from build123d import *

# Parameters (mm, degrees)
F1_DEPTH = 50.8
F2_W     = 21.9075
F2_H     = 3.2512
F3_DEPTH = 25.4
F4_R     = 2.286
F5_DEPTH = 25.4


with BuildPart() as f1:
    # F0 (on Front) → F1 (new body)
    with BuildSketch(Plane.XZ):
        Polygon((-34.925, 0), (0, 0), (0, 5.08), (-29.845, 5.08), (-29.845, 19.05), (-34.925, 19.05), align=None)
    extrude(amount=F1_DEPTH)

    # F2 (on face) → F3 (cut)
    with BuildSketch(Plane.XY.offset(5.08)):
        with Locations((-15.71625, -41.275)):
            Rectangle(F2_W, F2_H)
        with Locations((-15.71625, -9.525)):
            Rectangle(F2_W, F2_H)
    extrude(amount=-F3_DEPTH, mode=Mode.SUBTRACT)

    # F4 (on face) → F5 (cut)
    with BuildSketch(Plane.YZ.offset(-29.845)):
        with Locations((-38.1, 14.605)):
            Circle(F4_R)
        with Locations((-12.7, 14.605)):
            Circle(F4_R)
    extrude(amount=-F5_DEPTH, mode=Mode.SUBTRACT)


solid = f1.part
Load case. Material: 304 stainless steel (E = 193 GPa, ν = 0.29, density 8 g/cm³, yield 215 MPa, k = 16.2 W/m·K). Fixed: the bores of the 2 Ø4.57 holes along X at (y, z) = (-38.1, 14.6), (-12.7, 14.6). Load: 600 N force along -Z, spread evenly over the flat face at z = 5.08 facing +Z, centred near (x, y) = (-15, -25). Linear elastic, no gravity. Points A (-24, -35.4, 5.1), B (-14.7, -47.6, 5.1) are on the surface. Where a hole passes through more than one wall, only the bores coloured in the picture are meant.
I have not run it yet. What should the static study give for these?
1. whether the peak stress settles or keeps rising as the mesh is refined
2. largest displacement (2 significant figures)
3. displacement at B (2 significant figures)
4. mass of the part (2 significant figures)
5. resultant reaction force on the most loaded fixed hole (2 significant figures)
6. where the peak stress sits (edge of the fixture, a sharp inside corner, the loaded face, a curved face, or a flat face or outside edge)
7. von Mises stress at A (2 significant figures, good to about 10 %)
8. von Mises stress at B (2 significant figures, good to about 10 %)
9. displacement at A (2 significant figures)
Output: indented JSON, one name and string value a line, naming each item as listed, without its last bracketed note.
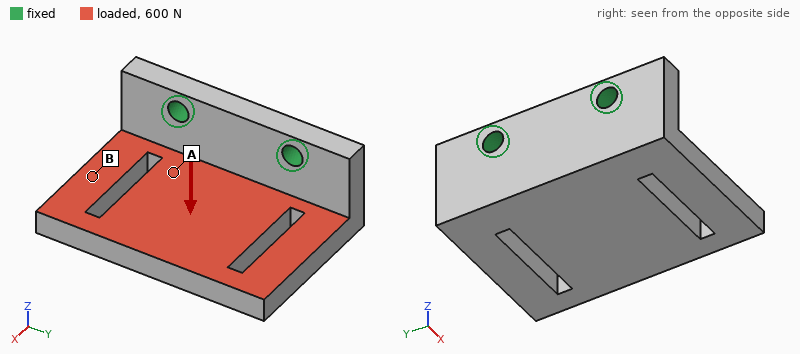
{
  "whether the peak stress settles or keeps rising as the mesh is refined": "keeps rising",
  "largest displacement": "65 µm",
  "displacement at B": "31 µm",
  "mass of the part": "94 g",
  "resultant reaction force on the most loaded fixed hole": "300 N",
  "where the peak stress sits": "edge of the fixture",
  "von Mises stress at A": "29 MPa",
  "von Mises stress at B": "12 MPa",
  "displacement at A": "13 µm"
}
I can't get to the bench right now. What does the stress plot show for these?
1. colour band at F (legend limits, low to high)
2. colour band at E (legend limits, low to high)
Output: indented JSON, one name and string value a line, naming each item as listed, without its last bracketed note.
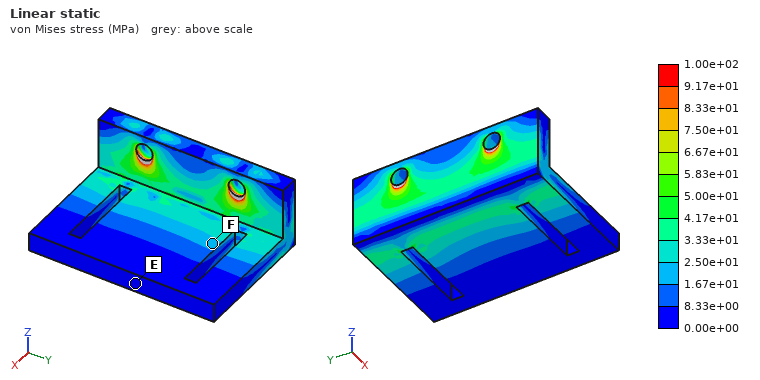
{
  "colour band at F": "1.67e+01 to 2.50e+01 MPa",
  "colour band at E": "0.00e+00 to 8.33e+00 MPa"
}
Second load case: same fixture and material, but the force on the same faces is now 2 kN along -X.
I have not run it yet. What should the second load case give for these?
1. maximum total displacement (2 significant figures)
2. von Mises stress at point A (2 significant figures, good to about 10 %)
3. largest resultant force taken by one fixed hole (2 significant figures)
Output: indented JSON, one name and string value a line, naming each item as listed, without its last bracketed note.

{
  "maximum total displacement": "20 µm",
  "von Mises stress at point A": "29 MPa",
  "largest resultant force taken by one fixed hole": "1.0 kN"
}
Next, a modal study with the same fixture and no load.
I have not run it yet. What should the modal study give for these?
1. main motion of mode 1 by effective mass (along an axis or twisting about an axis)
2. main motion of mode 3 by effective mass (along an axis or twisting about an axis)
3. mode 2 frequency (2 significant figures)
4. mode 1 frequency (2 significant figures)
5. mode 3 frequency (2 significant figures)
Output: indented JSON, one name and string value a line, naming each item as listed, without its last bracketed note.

{
  "main motion of mode 1 by effective mass": "along Z",
  "main motion of mode 3 by effective mass": "along Y",
  "mode 2 frequency": "4700 Hz",
  "mode 1 frequency": "2400 Hz",
  "mode 3 frequency": "6700 Hz"
}
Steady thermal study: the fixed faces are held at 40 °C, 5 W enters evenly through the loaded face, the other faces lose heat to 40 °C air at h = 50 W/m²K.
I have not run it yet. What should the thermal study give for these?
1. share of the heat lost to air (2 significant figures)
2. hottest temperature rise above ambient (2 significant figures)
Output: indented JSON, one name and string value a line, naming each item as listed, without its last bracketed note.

{
  "share of the heat lost to air": "51 %",
  "hottest temperature rise above ambient": "21 K"
}
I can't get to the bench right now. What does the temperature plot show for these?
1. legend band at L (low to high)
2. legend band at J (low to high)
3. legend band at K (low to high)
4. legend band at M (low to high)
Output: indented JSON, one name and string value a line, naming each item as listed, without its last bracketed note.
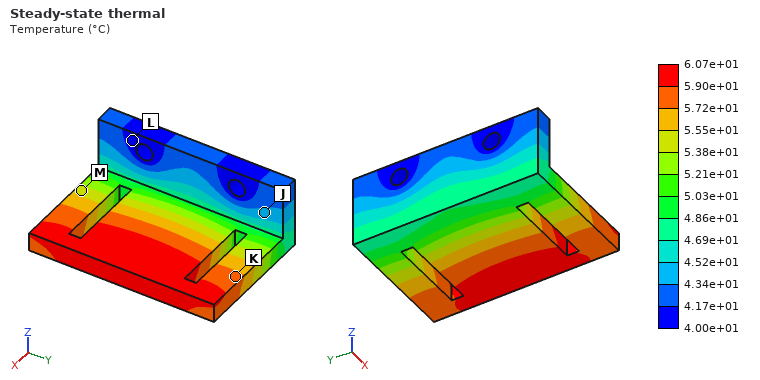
{
  "legend band at L": "4.00e+01 to 4.17e+01 °C",
  "legend band at J": "4.34e+01 to 4.52e+01 °C",
  "legend band at K": "5.72e+01 to 5.90e+01 °C",
  "legend band at M": "5.38e+01 to 5.55e+01 °C"
}
